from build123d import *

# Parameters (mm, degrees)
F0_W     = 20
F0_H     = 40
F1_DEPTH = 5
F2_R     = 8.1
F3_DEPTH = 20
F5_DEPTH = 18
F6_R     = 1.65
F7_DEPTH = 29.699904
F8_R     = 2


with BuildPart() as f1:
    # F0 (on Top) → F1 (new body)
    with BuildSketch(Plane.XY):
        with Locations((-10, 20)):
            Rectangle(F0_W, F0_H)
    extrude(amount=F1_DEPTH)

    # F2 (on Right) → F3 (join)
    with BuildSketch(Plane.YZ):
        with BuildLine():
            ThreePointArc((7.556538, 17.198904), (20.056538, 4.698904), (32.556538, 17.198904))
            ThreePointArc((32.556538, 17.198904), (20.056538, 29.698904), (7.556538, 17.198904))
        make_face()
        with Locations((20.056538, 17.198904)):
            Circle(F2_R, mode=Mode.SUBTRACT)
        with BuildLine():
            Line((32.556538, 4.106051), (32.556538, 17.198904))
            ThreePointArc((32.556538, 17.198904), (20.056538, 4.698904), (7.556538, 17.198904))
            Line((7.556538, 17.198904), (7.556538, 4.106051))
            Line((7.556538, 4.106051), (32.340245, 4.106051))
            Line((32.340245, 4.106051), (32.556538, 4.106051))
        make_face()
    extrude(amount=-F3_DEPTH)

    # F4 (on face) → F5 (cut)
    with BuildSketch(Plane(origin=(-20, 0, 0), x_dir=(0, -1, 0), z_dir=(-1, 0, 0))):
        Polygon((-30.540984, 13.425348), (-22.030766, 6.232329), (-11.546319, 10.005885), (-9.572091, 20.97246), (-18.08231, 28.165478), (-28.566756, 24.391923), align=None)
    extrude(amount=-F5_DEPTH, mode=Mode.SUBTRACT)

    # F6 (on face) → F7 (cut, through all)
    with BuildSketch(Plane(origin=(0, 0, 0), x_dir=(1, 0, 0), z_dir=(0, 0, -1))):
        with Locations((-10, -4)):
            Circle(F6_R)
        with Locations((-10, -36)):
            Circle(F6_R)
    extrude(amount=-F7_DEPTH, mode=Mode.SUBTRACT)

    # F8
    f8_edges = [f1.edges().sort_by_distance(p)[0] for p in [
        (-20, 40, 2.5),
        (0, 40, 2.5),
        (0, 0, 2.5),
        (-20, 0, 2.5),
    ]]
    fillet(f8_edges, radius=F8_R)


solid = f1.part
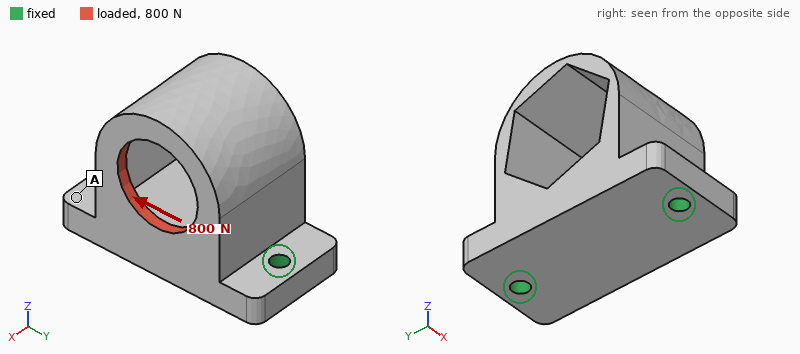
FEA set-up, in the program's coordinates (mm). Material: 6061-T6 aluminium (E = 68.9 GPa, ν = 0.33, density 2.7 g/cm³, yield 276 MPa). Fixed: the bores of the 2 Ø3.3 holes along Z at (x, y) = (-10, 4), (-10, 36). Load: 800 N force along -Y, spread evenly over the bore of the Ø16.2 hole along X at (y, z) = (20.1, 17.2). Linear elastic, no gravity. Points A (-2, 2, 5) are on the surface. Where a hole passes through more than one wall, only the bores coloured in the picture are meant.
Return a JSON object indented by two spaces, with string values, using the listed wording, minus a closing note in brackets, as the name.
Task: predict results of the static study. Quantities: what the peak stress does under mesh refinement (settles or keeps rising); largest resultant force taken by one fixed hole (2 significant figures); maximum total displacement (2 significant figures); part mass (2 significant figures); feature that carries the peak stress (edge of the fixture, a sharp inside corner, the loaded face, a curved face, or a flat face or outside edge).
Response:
{
  "what the peak stress does under mesh refinement": "keeps rising",
  "largest resultant force taken by one fixed hole": "620 N",
  "maximum total displacement": "32 µm",
  "part mass": "23 g",
  "feature that carries the peak stress": "a sharp inside corner"
}
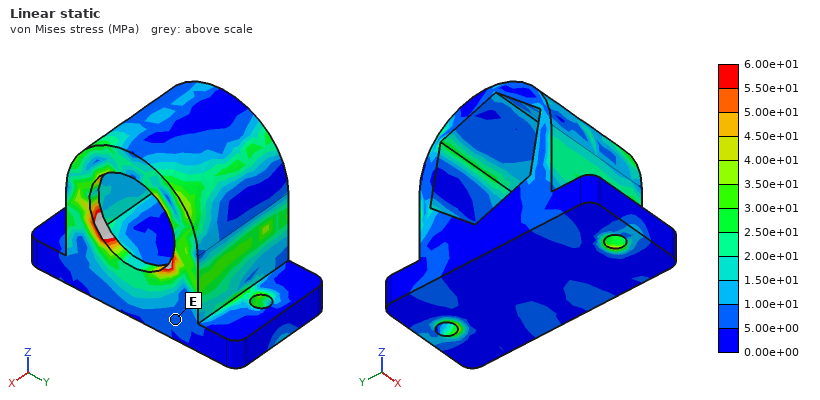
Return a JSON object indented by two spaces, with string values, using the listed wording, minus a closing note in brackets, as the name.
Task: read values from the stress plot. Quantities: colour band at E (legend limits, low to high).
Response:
{
  "colour band at E": "5.00e+00 to 1.00e+01 MPa"
}
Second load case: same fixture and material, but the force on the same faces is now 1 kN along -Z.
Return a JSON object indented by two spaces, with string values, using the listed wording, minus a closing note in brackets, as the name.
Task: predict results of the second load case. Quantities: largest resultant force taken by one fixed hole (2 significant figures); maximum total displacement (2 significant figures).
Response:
{
  "largest resultant force taken by one fixed hole": "530 N",
  "maximum total displacement": "53 µm"
}
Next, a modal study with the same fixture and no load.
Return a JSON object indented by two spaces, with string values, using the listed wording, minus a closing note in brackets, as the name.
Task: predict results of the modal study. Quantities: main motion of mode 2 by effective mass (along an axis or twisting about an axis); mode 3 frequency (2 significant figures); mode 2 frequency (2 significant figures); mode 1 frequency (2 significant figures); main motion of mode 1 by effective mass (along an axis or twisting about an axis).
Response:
{
  "main motion of mode 2 by effective mass": "along Y",
  "mode 3 frequency": "17 kHz",
  "mode 2 frequency": "8800 Hz",
  "mode 1 frequency": "6300 Hz",
  "main motion of mode 1 by effective mass": "along X"
}
